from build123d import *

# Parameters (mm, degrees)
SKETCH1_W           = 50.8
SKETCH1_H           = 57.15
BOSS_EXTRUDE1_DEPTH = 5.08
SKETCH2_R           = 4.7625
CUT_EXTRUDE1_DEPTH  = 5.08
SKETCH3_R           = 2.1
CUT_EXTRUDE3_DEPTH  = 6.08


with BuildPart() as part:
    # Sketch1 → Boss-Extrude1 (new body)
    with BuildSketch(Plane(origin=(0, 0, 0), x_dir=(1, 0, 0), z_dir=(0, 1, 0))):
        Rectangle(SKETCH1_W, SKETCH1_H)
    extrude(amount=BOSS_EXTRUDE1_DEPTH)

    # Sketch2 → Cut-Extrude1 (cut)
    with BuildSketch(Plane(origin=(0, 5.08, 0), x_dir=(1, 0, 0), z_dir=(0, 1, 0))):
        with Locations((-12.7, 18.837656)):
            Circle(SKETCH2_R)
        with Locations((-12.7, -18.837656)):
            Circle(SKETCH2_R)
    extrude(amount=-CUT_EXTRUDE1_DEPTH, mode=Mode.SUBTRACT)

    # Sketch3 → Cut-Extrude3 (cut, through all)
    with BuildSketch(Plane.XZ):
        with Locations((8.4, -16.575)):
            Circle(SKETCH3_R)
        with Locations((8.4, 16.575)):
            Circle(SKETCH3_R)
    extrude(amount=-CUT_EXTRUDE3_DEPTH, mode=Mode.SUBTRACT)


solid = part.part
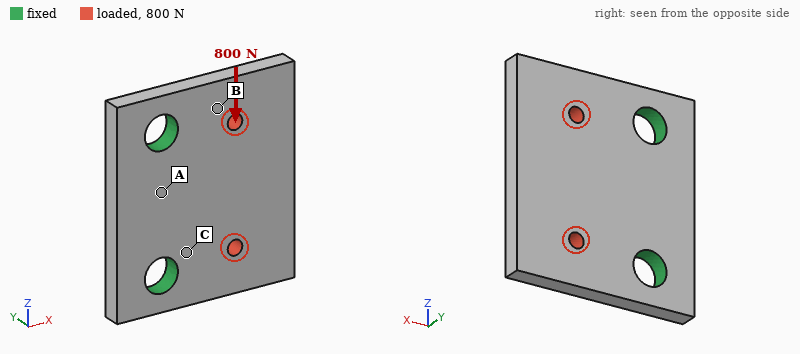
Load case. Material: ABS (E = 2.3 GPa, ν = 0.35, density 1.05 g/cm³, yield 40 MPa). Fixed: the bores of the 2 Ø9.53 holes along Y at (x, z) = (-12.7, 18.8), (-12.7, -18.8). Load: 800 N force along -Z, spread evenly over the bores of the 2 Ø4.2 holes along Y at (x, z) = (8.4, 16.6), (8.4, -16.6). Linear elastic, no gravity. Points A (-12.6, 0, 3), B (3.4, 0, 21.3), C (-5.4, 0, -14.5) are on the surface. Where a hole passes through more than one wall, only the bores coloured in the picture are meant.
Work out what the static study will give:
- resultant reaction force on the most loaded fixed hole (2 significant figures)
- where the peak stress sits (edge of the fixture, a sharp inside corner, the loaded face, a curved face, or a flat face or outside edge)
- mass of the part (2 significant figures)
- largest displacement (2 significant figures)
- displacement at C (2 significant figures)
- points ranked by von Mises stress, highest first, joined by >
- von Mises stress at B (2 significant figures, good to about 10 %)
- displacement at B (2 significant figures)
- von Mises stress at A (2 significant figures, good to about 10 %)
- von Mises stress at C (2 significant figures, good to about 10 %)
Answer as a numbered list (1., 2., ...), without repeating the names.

1. 530 N
2. edge of the fixture
3. 15 g
4. 0.11 mm
5. 0.019 mm
6. C > B > A
7. 4.6 MPa
8. 0.067 mm
9. 2.0 MPa
10. 6.7 MPa
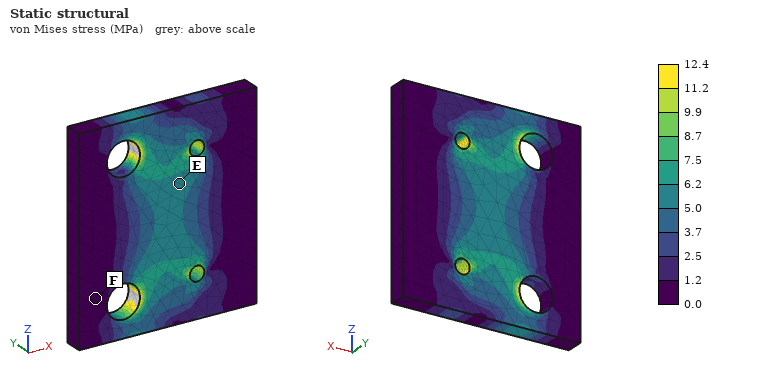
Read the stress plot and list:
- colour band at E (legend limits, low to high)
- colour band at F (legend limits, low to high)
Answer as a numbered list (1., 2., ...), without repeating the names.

1. 5.0 to 6.2 MPa
2. 0.0 to 1.2 MPa
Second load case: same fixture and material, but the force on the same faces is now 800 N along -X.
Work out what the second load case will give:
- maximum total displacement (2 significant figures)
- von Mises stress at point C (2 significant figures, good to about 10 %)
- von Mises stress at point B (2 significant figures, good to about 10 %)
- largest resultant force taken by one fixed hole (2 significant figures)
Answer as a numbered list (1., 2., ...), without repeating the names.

1. 42 µm
2. 4.2 MPa
3. 4.0 MPa
4. 400 N
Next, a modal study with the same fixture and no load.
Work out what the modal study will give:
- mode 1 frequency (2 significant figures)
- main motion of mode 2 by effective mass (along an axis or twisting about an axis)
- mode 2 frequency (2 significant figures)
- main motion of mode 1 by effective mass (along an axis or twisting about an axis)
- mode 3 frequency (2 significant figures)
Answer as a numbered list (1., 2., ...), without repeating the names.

1. 940 Hz
2. twisting about X
3. 1700 Hz
4. along Y
5. 3300 Hz
